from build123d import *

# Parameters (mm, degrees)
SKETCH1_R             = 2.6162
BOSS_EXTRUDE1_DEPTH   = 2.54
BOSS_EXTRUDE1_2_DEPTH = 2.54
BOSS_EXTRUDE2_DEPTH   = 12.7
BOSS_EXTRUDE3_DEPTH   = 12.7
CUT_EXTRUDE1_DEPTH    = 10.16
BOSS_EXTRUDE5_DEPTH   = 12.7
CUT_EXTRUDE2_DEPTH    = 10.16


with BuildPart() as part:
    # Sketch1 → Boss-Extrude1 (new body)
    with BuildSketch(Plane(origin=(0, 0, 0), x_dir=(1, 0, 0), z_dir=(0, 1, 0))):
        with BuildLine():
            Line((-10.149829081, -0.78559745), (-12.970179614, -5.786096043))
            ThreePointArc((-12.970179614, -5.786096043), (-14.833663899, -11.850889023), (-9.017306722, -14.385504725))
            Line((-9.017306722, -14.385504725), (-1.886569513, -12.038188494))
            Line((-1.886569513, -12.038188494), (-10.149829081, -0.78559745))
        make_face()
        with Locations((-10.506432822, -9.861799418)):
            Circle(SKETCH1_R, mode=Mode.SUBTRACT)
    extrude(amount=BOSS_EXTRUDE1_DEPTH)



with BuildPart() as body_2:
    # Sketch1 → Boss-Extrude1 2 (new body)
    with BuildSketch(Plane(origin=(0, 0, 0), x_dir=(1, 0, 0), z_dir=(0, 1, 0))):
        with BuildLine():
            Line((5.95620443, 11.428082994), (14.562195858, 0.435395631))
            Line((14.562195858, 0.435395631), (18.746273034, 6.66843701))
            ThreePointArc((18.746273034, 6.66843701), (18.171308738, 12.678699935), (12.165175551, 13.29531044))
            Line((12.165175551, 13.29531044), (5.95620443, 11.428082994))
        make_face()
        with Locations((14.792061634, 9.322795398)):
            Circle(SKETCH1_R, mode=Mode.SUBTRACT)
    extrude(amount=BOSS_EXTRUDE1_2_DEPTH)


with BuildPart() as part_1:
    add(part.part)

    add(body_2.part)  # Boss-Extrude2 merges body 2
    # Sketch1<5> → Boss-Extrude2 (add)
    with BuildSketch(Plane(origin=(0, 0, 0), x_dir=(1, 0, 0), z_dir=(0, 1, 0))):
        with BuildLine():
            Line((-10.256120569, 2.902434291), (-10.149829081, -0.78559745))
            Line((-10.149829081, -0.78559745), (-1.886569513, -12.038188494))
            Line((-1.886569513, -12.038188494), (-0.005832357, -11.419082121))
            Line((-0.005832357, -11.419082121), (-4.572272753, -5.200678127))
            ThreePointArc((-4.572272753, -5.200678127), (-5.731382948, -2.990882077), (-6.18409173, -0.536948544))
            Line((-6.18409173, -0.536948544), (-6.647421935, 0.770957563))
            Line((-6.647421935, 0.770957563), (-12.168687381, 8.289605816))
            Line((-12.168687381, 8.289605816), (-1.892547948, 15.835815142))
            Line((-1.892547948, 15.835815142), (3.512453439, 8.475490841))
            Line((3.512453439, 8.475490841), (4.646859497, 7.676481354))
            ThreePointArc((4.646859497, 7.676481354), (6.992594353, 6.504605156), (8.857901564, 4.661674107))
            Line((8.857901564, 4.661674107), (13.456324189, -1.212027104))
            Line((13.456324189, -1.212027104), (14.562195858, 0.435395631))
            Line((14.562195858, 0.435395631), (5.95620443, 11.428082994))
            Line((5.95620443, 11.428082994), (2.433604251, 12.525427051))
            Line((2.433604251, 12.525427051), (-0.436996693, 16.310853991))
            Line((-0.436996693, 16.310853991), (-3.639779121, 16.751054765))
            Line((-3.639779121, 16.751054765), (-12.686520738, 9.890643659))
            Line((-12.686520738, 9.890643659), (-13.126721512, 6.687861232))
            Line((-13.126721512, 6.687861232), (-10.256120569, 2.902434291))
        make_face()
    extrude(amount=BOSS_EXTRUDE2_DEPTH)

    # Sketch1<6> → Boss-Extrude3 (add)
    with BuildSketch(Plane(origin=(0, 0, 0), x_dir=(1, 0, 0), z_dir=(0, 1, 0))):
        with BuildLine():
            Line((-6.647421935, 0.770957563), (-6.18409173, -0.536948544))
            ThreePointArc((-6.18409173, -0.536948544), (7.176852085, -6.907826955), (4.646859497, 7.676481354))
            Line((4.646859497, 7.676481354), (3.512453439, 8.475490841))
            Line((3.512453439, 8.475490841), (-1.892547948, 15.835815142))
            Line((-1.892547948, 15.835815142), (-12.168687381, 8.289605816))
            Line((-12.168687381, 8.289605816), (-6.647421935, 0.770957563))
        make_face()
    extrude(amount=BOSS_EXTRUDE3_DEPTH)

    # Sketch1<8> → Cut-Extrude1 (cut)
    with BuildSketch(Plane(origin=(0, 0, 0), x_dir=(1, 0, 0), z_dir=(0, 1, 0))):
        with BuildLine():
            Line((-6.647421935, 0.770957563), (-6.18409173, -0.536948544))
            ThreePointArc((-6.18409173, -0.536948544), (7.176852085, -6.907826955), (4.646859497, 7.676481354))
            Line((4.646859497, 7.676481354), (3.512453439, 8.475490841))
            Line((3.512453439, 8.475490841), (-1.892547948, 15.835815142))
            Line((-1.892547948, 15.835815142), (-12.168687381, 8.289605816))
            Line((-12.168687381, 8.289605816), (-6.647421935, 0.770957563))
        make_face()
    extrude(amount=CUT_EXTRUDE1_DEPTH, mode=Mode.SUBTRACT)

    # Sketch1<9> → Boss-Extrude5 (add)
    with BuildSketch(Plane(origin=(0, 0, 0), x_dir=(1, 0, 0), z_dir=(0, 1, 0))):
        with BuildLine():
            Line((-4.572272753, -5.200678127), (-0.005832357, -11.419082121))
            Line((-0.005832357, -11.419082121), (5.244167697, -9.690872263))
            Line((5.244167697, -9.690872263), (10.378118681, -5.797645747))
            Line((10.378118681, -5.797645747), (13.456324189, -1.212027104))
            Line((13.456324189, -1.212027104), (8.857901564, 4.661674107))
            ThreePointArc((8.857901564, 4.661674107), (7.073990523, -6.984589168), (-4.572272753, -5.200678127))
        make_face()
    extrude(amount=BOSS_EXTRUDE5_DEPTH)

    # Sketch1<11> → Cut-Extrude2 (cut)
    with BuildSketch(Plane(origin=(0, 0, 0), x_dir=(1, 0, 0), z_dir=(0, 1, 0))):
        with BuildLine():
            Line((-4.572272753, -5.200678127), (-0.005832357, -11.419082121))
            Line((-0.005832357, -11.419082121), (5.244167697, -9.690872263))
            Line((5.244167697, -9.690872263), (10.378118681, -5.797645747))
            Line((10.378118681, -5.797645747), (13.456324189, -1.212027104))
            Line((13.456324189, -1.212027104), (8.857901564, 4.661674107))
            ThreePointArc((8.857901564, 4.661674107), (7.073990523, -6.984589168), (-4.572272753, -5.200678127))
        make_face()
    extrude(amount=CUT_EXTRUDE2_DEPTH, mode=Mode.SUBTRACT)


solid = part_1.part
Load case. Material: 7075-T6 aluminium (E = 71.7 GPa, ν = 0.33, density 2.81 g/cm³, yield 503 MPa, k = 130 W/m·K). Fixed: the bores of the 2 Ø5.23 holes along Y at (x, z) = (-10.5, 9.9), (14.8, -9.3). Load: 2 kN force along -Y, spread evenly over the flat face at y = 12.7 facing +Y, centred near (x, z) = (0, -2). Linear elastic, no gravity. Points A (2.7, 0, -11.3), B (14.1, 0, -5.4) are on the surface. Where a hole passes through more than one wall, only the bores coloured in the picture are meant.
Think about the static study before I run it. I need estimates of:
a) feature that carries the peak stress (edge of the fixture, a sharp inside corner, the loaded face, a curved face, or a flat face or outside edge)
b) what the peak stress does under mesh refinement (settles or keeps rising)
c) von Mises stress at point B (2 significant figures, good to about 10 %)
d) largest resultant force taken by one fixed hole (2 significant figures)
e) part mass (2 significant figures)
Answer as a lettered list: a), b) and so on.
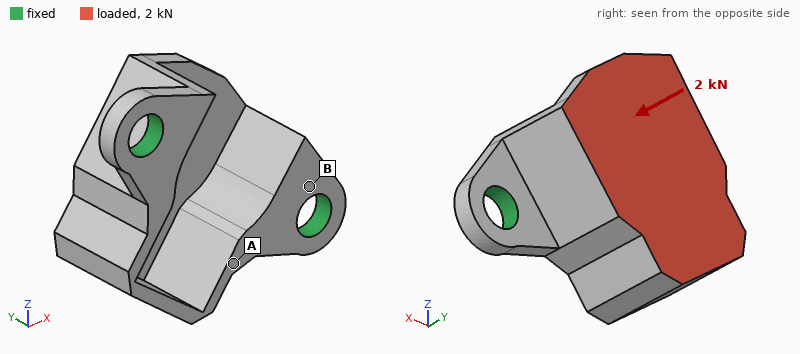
a) edge of the fixture
b) keeps rising
c) 97 MPa
d) 1.1 kN
e) 8.0 g
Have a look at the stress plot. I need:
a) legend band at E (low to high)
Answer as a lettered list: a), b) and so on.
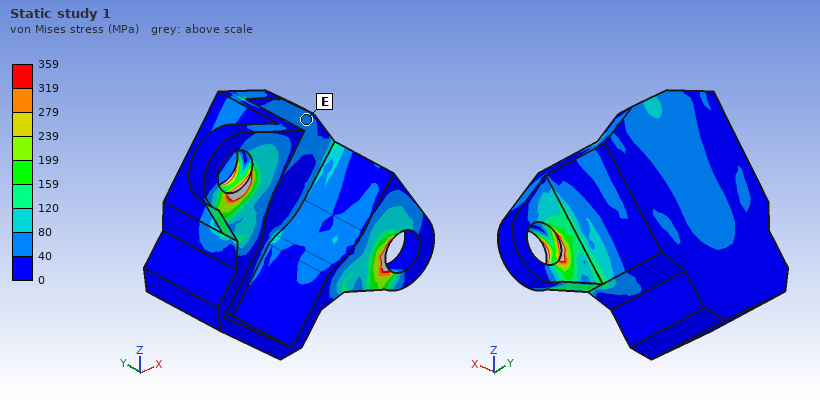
a) 40 to 80 MPa
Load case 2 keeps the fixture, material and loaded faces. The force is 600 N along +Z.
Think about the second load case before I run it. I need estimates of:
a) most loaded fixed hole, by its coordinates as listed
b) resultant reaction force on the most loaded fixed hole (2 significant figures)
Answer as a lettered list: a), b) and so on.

a) (-10.5, 9.9)
b) 350 N
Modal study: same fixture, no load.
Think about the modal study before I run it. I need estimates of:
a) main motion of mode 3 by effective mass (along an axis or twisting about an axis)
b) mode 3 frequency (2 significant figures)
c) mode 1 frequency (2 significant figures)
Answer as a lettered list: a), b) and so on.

a) twisting about Y
b) 11 kHz
c) 5100 Hz
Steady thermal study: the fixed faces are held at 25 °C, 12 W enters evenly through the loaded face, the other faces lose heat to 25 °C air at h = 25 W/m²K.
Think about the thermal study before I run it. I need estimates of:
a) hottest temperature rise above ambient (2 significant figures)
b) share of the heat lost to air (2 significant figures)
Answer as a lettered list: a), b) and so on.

a) 20 K
b) 6.1 %
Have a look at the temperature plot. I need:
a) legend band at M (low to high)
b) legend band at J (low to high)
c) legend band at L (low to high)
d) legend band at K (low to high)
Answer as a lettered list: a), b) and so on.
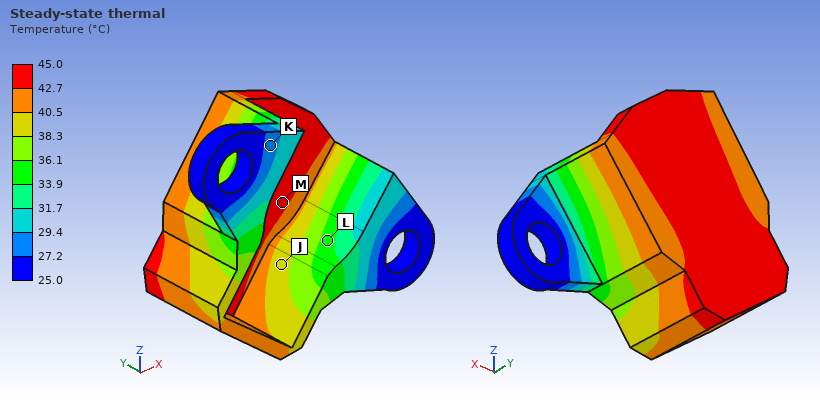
a) 42.7 to 45.0 °C
b) 38.3 to 40.5 °C
c) 33.9 to 36.1 °C
d) 27.2 to 29.4 °C
